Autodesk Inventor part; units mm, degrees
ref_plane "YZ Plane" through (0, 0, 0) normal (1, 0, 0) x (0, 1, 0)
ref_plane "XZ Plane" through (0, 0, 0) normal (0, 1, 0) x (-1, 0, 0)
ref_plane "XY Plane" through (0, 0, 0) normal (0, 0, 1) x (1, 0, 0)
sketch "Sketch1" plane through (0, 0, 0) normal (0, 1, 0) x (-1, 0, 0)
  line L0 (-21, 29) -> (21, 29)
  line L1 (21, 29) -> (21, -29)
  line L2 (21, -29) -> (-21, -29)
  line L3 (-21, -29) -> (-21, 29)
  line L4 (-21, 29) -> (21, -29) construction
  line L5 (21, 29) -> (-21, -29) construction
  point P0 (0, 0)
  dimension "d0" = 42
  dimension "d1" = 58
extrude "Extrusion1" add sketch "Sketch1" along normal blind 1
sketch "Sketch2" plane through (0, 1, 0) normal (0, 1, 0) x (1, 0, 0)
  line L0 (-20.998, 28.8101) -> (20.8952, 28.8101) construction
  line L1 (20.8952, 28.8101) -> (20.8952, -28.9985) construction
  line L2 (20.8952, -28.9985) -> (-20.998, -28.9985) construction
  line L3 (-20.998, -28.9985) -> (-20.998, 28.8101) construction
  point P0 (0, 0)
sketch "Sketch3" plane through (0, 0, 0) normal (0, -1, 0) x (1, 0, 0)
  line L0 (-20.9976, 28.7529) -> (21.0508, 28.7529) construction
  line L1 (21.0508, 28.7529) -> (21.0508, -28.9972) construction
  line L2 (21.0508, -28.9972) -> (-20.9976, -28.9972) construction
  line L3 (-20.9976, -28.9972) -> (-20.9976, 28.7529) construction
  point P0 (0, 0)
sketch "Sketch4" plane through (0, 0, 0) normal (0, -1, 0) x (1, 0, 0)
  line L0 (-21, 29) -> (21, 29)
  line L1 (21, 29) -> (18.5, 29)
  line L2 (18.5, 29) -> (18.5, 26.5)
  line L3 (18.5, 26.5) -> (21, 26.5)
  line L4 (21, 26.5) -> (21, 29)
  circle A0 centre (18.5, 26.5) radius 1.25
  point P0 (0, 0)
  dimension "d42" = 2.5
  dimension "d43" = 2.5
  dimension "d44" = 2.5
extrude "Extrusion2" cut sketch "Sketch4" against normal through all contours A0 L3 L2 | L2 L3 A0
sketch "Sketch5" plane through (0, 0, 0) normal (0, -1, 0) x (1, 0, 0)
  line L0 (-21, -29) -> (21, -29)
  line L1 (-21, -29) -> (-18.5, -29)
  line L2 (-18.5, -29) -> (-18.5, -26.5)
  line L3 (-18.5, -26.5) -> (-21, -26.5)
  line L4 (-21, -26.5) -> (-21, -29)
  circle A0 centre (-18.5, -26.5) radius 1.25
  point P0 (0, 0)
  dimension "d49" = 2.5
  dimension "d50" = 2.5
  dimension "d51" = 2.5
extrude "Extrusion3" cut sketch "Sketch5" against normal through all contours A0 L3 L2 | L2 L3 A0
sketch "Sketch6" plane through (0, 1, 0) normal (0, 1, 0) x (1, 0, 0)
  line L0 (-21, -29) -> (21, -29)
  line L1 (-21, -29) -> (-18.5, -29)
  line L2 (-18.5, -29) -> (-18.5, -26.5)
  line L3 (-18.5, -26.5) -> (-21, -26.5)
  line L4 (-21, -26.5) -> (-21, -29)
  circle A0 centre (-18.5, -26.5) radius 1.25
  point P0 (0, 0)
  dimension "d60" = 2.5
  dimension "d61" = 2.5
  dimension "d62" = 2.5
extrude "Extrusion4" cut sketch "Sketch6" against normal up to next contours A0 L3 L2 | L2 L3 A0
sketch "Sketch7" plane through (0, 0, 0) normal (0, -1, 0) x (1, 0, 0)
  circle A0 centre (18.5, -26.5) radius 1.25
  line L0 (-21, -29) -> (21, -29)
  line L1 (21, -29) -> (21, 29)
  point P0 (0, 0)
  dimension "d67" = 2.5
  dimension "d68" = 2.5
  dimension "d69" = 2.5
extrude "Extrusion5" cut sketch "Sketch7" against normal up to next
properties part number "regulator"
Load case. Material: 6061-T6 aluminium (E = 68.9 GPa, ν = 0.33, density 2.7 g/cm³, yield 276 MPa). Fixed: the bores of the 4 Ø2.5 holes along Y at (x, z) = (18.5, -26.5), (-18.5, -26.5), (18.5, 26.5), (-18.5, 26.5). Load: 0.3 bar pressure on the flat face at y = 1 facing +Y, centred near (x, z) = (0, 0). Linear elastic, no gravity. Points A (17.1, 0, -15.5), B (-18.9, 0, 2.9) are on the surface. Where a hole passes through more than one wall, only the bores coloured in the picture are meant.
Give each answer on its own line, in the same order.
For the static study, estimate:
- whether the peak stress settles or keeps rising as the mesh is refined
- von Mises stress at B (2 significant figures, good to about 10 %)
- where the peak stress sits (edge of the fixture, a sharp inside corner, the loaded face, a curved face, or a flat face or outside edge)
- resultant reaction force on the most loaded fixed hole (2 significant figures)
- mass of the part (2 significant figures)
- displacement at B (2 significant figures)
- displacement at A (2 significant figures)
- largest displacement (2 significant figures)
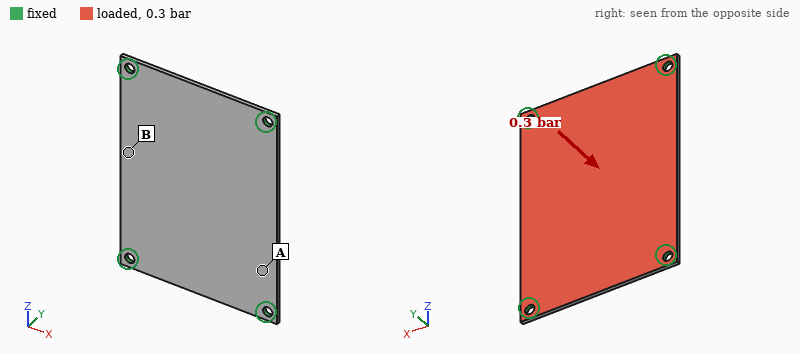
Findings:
keeps rising
27 MPa
edge of the fixture
18 N
6.5 g
0.14 mm
0.068 mm
0.17 mm
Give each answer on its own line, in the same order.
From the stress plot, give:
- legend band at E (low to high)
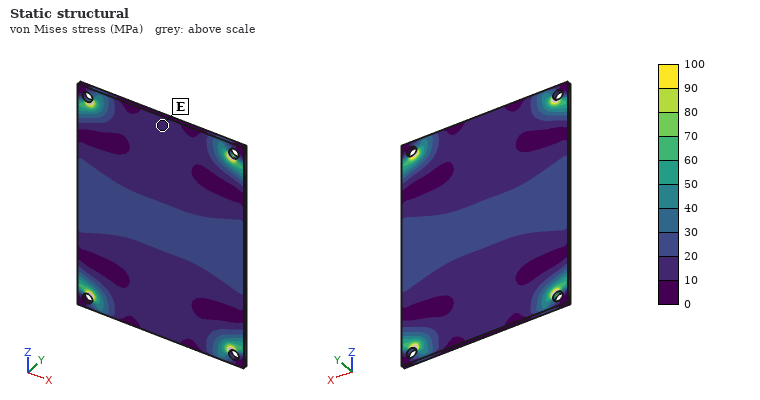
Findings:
10 to 20 MPa
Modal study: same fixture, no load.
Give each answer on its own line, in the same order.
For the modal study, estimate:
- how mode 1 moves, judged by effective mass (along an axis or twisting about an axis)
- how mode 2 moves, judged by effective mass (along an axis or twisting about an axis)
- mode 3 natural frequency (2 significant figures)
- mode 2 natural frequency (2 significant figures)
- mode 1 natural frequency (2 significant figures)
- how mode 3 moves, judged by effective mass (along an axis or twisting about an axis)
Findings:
along Y
twisting about Z
3600 Hz
2500 Hz
1500 Hz
twisting about X
